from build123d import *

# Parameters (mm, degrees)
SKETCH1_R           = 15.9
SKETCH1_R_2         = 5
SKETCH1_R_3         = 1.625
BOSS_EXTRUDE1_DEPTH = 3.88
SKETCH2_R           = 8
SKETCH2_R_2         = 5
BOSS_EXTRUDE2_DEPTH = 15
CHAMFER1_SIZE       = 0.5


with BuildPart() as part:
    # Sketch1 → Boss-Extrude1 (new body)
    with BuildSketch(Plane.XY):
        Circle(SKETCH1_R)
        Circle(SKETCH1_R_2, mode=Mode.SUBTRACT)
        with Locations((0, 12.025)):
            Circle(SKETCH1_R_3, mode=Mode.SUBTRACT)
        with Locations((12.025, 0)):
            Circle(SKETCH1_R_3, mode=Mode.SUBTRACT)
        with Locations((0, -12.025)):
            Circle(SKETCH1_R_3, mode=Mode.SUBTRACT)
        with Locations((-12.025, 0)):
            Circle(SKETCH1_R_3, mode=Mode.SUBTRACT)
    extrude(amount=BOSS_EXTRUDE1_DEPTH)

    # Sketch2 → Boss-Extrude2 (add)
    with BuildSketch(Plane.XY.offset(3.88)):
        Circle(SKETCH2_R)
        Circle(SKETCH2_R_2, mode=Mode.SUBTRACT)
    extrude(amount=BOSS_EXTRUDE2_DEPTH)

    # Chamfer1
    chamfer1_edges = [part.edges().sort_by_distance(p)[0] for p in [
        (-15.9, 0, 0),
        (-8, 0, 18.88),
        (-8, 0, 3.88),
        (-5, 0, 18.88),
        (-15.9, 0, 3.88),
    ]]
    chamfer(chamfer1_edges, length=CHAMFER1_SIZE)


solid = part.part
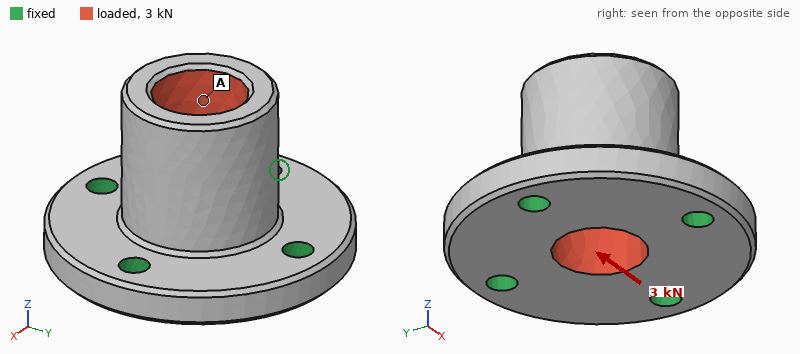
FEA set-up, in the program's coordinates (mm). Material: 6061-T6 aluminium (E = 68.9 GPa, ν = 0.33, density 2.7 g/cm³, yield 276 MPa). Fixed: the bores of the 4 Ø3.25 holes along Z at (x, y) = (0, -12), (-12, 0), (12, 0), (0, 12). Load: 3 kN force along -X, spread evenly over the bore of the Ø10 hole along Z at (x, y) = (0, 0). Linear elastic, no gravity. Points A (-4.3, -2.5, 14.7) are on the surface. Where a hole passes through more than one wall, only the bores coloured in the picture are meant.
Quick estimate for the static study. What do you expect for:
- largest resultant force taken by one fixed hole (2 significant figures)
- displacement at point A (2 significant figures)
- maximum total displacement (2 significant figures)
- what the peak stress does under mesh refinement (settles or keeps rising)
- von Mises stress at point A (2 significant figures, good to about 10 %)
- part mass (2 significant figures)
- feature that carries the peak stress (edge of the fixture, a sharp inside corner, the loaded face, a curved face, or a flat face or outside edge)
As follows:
1.4 kN
24 µm
31 µm
keeps rising
18 MPa
12 g
edge of the fixture
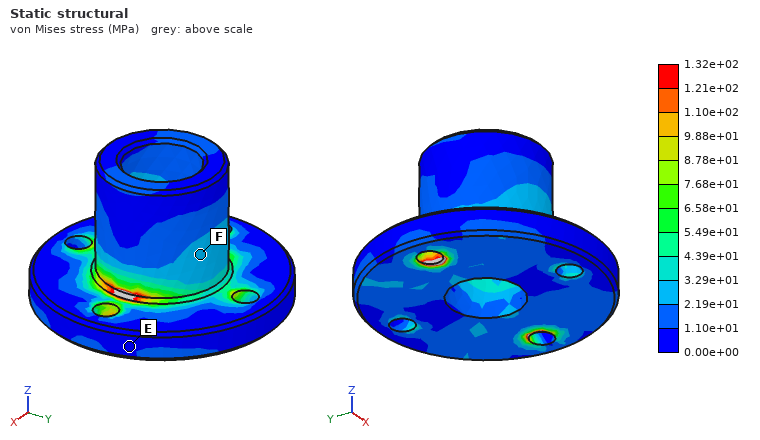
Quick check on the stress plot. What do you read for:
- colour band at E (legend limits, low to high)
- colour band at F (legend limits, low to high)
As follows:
0.00e+00 to 1.10e+01 MPa
2.19e+01 to 3.29e+01 MPa
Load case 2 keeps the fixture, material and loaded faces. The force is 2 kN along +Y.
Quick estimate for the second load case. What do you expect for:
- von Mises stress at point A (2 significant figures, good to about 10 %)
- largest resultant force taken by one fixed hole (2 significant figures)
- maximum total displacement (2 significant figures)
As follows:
15 MPa
910 N
21 µm
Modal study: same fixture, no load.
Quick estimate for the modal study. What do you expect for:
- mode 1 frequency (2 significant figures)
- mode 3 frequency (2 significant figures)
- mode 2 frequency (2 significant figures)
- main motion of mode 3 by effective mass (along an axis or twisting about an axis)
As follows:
22 kHz
37 kHz
23 kHz
along Z
